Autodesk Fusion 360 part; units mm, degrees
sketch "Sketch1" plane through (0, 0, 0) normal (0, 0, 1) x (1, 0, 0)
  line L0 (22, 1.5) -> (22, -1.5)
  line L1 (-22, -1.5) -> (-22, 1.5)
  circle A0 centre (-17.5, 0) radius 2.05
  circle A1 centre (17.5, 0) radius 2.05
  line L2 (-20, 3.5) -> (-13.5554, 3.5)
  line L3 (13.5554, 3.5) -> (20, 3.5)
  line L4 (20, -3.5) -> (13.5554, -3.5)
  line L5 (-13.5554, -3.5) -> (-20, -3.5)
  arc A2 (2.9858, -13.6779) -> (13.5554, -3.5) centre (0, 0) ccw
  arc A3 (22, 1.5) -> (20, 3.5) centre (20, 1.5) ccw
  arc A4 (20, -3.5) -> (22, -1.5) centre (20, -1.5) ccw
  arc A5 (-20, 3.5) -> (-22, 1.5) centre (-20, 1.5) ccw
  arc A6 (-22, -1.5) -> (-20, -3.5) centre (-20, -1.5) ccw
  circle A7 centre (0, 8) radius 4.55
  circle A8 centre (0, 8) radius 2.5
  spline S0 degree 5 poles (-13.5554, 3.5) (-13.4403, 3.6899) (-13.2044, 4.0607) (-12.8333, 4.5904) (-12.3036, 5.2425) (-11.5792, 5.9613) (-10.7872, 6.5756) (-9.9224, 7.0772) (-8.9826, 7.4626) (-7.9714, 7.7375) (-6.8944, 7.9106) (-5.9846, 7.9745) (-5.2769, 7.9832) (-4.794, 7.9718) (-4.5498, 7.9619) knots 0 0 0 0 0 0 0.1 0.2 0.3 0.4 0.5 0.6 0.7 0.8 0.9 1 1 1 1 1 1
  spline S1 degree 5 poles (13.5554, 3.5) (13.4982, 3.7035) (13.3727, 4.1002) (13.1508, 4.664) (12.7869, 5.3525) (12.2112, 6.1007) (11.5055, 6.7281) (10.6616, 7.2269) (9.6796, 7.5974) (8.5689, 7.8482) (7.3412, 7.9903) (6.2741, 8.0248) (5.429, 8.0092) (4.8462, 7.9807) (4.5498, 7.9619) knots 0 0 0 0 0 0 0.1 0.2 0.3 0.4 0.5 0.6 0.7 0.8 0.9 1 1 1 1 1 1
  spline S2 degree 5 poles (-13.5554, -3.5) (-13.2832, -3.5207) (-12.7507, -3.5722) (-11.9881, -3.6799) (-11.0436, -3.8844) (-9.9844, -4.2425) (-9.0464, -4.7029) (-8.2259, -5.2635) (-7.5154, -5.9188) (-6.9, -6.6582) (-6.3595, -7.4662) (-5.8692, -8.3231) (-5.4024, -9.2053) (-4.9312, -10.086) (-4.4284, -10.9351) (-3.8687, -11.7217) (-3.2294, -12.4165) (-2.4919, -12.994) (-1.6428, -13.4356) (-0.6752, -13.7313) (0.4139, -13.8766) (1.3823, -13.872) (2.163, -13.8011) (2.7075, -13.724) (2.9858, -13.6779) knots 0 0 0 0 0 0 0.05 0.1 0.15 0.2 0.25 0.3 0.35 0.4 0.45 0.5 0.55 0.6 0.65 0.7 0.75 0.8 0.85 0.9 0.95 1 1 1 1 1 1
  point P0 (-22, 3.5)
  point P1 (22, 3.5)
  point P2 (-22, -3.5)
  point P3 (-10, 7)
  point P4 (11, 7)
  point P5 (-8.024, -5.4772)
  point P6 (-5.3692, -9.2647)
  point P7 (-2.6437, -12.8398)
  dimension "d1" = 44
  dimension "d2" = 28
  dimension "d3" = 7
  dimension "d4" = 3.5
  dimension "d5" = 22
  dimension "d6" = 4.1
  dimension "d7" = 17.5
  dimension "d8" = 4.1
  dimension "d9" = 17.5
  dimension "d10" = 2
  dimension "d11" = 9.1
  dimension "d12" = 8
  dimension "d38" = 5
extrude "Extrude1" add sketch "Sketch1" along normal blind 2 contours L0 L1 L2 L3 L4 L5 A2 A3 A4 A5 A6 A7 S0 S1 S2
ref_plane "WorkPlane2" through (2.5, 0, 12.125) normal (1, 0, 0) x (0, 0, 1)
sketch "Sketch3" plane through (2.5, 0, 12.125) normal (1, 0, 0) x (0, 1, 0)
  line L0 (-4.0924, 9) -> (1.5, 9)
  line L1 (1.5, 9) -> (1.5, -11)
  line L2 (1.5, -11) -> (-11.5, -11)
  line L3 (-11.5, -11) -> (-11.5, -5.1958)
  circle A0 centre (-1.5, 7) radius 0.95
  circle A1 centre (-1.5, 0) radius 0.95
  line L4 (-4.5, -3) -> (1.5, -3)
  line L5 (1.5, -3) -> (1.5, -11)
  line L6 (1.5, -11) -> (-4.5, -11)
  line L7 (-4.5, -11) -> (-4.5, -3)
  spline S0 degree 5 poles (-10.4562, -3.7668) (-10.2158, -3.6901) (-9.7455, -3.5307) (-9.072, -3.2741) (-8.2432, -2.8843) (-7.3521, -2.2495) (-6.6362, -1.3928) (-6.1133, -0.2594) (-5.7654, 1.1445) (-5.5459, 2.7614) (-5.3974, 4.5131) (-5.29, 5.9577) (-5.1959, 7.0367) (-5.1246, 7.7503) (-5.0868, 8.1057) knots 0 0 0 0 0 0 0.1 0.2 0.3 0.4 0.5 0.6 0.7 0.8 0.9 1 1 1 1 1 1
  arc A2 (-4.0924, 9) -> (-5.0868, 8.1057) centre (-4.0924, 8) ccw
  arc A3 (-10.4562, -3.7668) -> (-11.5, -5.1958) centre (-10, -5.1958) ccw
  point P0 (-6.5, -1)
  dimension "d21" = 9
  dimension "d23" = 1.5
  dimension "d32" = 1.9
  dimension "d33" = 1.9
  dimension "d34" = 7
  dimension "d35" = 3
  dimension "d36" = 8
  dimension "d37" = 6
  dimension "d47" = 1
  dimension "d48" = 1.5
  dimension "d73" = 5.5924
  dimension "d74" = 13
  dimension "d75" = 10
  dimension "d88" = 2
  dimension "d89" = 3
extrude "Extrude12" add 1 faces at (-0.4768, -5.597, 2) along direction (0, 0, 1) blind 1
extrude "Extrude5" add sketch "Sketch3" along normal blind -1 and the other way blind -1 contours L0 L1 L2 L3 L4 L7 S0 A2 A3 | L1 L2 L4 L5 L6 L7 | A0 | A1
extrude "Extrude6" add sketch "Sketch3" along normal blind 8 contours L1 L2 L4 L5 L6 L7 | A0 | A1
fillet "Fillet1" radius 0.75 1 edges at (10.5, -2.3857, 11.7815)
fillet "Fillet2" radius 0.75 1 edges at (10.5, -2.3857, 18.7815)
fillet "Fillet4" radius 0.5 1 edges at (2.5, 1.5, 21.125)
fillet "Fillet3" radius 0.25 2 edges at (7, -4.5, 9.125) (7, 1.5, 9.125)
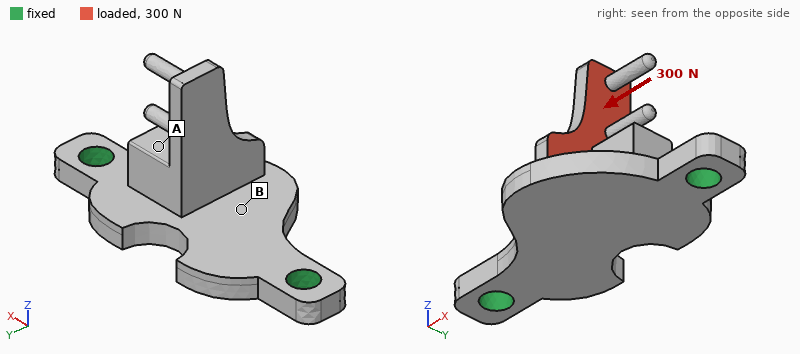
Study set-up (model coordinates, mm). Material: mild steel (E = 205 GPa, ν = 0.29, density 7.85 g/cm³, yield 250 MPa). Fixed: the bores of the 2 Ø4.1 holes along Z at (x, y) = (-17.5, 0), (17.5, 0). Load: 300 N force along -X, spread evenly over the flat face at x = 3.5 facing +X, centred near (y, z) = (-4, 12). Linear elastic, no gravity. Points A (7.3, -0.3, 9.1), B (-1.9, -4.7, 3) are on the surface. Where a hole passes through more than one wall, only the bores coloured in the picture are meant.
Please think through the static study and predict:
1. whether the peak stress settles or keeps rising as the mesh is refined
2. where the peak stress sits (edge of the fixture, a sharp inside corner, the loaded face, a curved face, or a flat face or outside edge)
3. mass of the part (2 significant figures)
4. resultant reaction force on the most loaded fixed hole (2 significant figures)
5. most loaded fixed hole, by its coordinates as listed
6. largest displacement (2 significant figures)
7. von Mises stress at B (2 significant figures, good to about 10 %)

keeps rising
a sharp inside corner
17 g
230 N
(17.5, 0)
76 µm
44 MPa
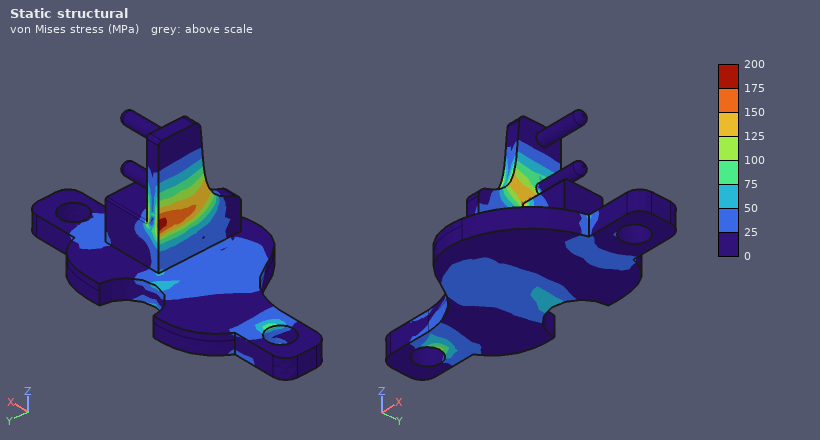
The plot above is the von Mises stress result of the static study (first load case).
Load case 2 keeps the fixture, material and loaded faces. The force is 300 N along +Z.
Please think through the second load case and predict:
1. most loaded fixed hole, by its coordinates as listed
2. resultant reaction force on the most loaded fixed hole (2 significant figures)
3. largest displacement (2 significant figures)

(17.5, 0)
190 N
23 µm
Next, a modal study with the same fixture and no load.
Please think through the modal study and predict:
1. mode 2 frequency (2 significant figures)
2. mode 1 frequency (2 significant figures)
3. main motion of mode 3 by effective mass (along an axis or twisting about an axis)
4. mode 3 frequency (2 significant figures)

7300 Hz
5900 Hz
along Z
10 kHz
